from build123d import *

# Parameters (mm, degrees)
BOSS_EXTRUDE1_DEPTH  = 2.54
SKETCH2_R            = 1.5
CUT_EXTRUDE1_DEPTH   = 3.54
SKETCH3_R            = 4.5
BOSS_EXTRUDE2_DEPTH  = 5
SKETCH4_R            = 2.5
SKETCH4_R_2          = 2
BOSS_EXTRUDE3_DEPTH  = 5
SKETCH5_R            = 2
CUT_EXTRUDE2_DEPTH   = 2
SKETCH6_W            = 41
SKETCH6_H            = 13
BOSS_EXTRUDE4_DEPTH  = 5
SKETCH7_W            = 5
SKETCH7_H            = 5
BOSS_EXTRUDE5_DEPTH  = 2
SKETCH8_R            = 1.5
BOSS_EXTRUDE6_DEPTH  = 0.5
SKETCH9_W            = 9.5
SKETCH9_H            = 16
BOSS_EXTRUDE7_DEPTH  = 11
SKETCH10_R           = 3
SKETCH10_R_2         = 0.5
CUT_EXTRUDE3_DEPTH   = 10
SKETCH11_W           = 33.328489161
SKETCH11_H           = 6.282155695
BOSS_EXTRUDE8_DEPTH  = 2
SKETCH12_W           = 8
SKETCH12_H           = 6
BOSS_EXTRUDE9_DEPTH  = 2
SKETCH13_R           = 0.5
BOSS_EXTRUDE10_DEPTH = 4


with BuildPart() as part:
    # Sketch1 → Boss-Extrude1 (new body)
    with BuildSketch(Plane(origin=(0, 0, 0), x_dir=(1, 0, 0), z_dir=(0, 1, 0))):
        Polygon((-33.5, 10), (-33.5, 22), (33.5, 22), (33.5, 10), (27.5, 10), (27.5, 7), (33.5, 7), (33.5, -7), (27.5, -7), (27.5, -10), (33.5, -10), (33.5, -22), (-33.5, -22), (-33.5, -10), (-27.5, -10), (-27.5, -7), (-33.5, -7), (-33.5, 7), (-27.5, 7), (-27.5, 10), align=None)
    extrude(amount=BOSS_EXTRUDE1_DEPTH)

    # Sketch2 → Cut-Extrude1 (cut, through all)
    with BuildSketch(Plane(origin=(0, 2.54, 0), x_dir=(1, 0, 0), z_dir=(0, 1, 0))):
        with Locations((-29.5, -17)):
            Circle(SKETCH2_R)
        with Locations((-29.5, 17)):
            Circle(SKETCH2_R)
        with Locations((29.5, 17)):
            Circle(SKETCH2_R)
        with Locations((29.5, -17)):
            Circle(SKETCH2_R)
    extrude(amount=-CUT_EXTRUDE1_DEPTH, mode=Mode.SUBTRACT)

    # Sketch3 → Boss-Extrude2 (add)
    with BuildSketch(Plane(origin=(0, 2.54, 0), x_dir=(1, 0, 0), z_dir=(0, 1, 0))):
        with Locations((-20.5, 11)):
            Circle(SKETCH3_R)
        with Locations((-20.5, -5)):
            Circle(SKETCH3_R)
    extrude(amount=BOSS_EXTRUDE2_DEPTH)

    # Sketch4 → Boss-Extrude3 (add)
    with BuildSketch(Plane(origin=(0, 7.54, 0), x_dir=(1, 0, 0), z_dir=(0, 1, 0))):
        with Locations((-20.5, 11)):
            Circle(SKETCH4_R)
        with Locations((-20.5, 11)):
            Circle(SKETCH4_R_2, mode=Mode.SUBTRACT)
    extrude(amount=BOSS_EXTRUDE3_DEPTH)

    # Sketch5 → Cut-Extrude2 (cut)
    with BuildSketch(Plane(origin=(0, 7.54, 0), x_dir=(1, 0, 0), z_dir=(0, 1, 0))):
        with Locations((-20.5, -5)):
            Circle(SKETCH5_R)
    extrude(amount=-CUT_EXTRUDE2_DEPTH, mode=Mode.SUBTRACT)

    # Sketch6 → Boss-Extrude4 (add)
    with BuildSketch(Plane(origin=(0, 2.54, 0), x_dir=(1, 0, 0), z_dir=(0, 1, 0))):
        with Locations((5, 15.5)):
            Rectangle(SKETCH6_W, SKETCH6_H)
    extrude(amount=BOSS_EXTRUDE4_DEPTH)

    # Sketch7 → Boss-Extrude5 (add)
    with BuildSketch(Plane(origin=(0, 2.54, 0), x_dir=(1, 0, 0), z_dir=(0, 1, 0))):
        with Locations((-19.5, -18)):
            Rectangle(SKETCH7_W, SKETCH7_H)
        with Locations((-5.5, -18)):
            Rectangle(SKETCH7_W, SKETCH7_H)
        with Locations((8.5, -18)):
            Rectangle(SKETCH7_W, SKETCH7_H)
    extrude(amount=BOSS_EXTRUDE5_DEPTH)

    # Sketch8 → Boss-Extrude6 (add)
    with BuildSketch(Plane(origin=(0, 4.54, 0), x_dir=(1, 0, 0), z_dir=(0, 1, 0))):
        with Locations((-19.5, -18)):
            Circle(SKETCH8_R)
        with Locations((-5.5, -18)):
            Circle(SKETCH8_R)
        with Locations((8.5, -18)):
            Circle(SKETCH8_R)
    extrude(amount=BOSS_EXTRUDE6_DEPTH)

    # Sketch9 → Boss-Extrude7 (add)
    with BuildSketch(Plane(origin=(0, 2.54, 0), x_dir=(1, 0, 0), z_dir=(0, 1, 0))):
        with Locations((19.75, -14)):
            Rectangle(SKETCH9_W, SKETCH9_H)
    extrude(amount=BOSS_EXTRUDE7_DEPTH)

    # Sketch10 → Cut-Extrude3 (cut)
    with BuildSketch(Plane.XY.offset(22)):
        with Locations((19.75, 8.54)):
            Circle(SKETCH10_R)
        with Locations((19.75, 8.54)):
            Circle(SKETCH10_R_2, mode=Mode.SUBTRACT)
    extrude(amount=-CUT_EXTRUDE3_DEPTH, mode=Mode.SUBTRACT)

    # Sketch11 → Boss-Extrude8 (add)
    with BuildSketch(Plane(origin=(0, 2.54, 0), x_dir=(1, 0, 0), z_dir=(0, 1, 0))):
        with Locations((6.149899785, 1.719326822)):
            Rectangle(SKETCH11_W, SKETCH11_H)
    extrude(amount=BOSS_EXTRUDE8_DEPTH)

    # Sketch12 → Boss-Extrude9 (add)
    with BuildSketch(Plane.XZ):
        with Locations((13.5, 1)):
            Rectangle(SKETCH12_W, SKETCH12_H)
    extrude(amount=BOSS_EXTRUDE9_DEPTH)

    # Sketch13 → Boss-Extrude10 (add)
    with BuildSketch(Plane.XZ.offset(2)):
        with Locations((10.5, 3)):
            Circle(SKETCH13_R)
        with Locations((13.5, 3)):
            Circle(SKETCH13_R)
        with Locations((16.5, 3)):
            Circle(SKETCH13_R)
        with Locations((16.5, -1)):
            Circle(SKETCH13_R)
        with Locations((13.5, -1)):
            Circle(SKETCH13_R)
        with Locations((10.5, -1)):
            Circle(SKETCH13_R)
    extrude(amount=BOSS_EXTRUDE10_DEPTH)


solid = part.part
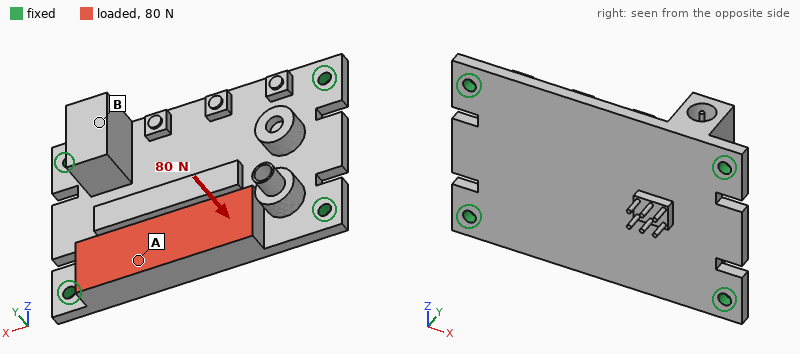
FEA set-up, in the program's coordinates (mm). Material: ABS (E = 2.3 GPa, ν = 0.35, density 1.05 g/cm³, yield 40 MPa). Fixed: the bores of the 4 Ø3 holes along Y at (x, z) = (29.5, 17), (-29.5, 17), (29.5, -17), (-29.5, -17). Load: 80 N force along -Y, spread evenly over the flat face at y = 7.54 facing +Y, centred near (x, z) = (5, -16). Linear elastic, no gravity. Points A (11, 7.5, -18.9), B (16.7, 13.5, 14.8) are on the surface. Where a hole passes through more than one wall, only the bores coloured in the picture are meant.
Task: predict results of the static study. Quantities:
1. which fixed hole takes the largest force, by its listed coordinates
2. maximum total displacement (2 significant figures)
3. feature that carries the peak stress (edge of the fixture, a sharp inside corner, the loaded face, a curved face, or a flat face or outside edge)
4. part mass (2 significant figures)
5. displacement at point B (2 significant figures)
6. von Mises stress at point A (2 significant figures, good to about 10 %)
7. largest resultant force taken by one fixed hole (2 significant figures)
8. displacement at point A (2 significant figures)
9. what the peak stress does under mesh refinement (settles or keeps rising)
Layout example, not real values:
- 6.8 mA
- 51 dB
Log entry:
- (29.5, -17)
- 0.20 mm
- edge of the fixture
- 13 g
- 0.064 mm
- 2.7 MPa
- 65 N
- 0.14 mm
- keeps rising
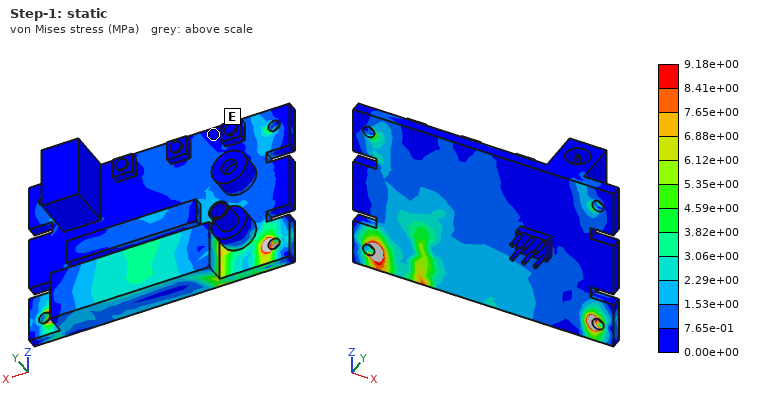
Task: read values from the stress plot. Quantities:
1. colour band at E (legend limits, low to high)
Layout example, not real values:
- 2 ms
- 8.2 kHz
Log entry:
- 0.00e+00 to 7.65e-01 MPa
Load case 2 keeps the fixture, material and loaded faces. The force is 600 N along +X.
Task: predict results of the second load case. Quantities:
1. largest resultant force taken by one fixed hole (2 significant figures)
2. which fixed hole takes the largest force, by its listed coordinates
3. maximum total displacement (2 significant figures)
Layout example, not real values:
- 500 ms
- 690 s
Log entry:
- 280 N
- (29.5, -17)
- 0.35 mm
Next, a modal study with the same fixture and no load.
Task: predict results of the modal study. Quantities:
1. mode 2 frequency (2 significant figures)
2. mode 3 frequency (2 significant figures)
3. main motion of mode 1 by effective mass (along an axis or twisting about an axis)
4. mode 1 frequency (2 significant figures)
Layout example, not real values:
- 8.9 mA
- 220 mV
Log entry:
- 1700 Hz
- 2000 Hz
- along Y
- 1100 Hz
